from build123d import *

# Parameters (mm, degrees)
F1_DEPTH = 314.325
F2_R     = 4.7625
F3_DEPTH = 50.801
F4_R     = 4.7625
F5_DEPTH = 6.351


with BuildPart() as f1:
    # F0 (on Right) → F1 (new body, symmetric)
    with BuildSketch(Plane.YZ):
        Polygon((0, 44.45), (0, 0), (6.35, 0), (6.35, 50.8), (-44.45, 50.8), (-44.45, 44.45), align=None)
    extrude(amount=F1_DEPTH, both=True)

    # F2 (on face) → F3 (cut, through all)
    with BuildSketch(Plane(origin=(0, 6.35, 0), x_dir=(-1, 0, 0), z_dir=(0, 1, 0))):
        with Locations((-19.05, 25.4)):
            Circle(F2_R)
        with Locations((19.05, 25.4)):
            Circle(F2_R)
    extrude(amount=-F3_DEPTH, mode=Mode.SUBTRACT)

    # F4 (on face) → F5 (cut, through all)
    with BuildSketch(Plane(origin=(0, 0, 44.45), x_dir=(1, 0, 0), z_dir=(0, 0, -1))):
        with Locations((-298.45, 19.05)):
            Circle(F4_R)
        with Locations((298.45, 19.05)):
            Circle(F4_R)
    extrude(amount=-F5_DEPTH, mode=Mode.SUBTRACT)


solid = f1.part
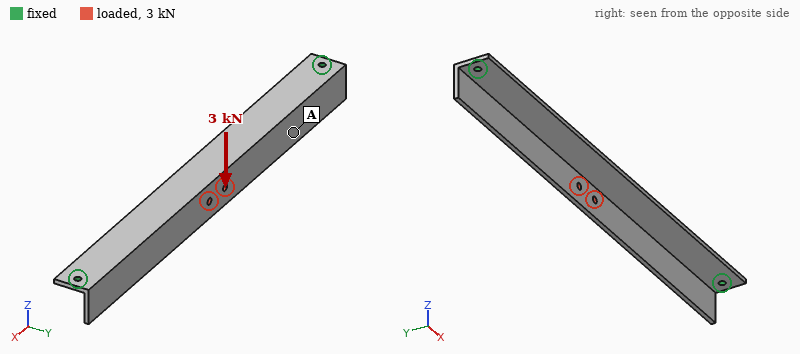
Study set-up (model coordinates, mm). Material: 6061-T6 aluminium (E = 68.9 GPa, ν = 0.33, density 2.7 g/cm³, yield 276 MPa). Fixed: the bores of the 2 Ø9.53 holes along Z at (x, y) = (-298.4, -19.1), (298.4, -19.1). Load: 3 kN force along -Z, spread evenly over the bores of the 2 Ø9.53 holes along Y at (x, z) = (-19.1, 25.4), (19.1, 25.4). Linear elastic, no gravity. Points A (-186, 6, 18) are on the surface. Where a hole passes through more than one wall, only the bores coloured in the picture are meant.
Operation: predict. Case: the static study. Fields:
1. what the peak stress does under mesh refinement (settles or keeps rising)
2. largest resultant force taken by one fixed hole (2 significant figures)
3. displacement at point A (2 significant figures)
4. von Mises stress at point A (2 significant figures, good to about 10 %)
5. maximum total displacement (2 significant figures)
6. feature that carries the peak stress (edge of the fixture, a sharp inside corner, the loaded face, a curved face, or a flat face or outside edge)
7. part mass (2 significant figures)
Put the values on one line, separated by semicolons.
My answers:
keeps rising; 5.1 kN; 0.86 mm; 20 MPa; 1.7 mm; edge of the fixture; 1.0 kg
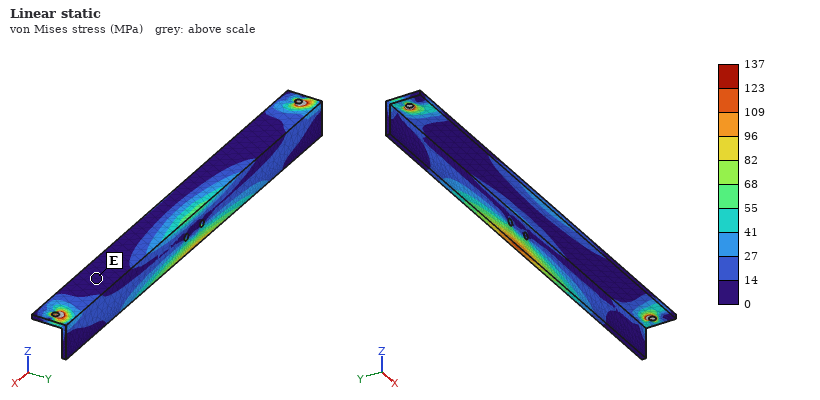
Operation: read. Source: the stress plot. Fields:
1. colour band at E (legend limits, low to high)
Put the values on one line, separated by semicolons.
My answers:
0 to 14 MPa
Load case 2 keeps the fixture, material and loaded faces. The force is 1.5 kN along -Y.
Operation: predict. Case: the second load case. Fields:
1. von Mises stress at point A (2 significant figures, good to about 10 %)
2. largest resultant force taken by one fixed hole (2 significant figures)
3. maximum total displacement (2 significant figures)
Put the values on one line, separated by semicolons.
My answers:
23 MPa; 870 N; 1.7 mm
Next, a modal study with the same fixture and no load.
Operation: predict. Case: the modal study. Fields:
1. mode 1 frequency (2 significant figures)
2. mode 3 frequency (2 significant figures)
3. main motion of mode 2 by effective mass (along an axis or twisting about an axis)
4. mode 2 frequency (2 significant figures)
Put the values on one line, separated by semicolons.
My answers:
310 Hz; 660 Hz; along Z; 330 Hz
